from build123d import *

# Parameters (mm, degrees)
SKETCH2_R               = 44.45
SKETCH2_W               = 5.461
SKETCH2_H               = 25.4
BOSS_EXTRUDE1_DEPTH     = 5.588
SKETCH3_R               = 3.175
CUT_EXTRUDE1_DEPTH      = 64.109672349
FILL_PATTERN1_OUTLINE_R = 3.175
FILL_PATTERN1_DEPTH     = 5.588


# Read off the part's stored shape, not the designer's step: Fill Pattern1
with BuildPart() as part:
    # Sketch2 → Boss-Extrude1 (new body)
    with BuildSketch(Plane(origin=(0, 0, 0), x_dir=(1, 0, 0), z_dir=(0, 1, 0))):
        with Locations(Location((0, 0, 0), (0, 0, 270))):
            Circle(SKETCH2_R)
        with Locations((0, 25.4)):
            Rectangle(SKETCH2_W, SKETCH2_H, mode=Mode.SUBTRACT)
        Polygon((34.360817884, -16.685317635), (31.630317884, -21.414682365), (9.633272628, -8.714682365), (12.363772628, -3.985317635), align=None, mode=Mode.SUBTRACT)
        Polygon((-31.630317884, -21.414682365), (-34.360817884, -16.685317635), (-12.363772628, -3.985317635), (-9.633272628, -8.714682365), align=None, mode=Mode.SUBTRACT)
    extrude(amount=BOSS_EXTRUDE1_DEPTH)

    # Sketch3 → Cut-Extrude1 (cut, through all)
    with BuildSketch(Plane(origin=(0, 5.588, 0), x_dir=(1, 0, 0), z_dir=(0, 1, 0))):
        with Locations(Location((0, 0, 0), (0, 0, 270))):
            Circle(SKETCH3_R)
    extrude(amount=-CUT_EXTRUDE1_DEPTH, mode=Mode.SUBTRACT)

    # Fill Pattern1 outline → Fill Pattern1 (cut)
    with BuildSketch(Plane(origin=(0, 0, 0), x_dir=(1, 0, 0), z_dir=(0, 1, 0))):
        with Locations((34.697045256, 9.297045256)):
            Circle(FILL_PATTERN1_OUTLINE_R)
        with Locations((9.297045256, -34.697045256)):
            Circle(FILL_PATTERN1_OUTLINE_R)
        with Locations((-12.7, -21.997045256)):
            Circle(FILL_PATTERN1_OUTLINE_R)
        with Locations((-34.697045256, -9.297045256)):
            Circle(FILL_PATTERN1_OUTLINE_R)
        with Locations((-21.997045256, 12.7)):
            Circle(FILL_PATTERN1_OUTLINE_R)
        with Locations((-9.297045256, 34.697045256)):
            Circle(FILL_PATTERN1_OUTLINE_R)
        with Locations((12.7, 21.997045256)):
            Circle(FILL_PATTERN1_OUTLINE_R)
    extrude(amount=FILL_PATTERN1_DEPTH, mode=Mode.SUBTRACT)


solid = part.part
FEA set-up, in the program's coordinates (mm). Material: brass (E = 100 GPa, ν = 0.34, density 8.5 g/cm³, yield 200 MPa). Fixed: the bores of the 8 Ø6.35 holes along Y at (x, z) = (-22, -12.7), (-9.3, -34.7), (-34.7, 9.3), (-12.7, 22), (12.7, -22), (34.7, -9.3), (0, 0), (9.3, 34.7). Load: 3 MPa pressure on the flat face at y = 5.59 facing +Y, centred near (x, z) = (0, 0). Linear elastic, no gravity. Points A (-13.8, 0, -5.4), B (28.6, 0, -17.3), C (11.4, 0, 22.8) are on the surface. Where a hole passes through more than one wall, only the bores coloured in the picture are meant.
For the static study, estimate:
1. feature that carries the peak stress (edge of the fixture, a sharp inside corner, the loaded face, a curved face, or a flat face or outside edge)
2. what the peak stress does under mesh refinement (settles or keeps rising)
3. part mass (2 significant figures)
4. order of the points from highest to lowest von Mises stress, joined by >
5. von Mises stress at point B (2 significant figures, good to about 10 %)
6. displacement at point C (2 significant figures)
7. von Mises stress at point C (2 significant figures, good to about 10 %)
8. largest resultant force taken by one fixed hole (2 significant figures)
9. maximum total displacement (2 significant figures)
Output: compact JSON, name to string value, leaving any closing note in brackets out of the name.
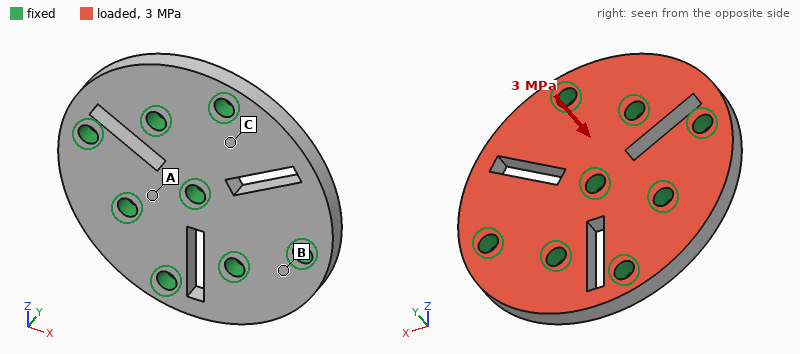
{"feature that carries the peak stress": "edge of the fixture", "what the peak stress does under mesh refinement": "keeps rising", "part mass": "260 g", "order of the points from highest to lowest von Mises stress, joined by >": "C > B > A", "von Mises stress at point B": "29 MPa", "displacement at point C": "14 µm", "von Mises stress at point C": "42 MPa", "largest resultant force taken by one fixed hole": "2.6 kN", "maximum total displacement": "76 µm"}
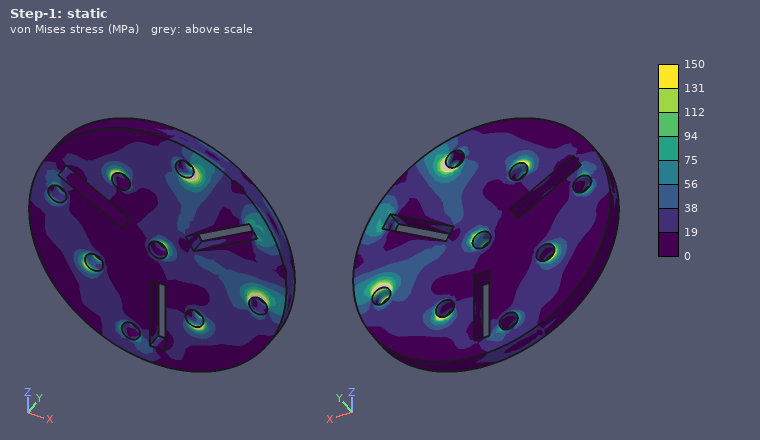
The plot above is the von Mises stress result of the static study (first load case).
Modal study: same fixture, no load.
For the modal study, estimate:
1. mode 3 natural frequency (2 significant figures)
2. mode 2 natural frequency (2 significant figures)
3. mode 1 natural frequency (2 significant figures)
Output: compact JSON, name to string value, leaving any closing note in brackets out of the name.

{"mode 3 natural frequency": "10 kHz", "mode 2 natural frequency": "10 kHz", "mode 1 natural frequency": "6100 Hz"}
